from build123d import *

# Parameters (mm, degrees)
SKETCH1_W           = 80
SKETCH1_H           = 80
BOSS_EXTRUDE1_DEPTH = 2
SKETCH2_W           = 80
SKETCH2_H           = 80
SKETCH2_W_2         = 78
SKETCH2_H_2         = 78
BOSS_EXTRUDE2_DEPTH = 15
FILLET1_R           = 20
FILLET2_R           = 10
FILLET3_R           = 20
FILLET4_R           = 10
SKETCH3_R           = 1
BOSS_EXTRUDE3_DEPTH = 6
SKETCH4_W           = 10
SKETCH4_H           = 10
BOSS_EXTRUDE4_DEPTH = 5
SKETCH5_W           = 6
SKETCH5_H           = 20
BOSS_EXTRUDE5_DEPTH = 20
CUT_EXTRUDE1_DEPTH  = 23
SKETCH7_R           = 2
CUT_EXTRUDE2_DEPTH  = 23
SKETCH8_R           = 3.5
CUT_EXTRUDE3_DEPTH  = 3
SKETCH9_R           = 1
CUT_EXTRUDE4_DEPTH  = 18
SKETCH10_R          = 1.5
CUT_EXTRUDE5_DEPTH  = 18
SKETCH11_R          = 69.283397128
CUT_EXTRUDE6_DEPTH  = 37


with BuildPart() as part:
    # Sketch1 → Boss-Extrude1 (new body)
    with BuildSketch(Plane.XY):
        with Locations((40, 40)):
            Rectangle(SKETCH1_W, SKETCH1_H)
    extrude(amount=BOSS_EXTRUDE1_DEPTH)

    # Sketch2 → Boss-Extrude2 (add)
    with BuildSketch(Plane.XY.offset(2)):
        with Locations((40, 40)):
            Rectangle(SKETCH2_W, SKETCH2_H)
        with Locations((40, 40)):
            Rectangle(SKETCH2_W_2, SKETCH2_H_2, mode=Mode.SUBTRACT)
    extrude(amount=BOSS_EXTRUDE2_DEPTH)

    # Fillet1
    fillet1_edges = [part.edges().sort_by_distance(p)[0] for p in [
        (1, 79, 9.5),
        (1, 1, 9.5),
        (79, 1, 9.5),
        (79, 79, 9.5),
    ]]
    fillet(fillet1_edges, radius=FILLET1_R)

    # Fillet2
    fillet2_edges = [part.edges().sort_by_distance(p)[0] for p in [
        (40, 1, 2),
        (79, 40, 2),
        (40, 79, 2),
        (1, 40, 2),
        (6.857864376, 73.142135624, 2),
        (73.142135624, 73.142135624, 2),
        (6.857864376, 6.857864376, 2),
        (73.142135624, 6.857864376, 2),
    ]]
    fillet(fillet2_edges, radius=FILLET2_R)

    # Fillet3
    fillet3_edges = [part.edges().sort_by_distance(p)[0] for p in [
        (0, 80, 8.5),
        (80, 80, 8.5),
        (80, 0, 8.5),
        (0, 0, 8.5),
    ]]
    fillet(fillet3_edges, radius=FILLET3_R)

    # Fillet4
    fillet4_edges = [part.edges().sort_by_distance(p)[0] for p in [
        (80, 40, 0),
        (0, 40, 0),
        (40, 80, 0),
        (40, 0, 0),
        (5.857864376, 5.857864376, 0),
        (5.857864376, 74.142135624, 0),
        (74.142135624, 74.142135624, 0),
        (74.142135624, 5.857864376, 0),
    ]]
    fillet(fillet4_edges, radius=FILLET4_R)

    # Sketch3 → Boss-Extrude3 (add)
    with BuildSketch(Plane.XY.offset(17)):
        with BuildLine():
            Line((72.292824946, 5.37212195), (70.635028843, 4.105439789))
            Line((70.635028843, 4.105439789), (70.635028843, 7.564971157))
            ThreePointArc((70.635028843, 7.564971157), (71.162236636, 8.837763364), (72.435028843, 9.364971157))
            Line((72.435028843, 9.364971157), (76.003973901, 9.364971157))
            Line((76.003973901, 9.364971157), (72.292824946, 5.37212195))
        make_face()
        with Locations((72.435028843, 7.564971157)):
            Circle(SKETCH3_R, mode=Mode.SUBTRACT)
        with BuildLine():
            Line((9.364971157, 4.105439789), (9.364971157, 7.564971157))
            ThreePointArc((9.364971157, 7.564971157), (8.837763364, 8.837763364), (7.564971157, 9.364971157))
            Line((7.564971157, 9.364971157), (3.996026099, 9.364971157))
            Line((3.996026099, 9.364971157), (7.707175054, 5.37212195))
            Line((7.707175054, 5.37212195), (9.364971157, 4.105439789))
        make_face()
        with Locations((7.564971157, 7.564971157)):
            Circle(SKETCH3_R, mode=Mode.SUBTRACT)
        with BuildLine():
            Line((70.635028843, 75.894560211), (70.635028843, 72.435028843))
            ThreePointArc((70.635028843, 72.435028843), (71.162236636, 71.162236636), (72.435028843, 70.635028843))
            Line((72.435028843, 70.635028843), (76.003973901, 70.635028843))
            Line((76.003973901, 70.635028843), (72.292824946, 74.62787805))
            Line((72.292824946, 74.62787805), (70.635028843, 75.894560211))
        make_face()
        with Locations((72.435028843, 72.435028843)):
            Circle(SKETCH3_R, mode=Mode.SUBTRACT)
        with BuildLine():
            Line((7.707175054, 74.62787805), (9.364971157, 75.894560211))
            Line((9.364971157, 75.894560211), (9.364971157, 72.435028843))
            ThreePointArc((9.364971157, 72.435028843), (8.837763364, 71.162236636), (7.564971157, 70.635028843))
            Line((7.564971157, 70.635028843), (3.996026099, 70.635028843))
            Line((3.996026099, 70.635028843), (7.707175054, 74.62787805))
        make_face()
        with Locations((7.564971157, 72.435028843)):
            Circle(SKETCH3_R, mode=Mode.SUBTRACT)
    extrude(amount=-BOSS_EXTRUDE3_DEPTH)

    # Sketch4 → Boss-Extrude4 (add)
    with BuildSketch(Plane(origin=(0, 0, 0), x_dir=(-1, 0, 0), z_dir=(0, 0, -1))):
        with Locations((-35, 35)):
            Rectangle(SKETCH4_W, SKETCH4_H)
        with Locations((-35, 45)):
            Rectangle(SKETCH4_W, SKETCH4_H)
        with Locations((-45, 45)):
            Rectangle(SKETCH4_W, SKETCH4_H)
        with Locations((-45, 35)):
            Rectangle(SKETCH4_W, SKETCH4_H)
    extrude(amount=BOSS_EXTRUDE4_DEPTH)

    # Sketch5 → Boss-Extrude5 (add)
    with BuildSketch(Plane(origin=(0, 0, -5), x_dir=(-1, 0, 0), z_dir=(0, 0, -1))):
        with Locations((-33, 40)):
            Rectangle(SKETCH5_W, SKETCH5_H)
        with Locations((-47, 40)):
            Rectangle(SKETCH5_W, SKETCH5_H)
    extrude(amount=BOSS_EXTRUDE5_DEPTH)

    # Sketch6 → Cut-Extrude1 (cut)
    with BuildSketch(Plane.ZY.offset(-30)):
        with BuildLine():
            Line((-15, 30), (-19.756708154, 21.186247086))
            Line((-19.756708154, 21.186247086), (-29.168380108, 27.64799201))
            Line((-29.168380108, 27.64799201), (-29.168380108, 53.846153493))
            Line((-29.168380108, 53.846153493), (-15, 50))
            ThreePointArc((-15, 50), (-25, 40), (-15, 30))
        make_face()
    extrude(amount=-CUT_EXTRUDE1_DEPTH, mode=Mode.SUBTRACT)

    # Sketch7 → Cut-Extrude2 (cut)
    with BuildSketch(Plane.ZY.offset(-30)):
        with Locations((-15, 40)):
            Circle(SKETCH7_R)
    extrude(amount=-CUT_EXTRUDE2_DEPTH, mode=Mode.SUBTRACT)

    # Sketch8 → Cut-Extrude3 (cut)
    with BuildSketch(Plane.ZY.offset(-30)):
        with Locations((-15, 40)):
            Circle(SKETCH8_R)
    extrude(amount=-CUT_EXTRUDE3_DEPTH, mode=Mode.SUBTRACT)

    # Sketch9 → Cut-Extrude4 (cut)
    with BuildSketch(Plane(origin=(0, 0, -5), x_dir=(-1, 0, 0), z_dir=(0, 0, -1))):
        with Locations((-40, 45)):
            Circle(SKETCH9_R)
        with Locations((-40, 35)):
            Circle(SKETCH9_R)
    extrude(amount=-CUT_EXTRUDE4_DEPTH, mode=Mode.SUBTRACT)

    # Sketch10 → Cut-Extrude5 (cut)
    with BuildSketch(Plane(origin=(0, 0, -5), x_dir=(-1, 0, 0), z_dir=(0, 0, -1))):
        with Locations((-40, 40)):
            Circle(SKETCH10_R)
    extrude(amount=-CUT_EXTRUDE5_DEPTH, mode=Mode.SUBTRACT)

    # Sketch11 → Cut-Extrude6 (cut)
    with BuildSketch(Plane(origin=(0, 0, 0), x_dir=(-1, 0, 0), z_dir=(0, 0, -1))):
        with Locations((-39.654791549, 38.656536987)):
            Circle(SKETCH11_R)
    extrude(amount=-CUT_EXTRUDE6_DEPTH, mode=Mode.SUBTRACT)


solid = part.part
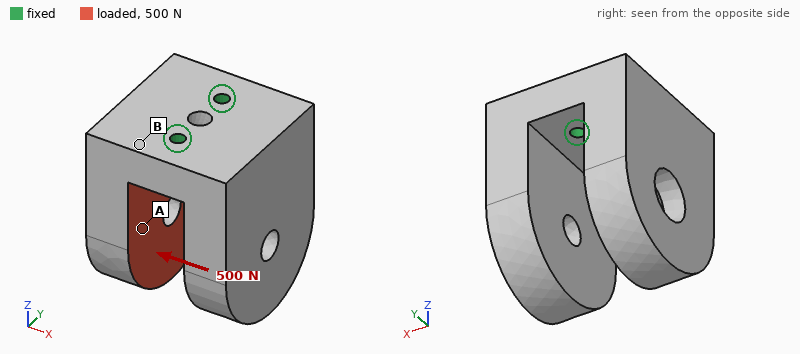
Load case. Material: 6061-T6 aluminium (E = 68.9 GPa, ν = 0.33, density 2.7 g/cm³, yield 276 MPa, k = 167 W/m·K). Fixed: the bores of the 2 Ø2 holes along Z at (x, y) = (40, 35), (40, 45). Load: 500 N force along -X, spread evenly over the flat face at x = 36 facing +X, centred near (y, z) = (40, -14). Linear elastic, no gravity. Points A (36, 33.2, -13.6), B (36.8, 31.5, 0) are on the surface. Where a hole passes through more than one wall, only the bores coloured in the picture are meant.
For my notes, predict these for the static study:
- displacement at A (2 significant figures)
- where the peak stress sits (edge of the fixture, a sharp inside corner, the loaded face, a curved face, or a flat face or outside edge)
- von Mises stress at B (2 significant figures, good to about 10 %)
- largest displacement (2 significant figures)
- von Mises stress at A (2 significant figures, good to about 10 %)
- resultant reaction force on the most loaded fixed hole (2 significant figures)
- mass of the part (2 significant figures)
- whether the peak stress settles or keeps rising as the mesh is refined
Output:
39 µm
edge of the fixture
54 MPa
91 µm
14 MPa
260 N
16 g
keeps rising
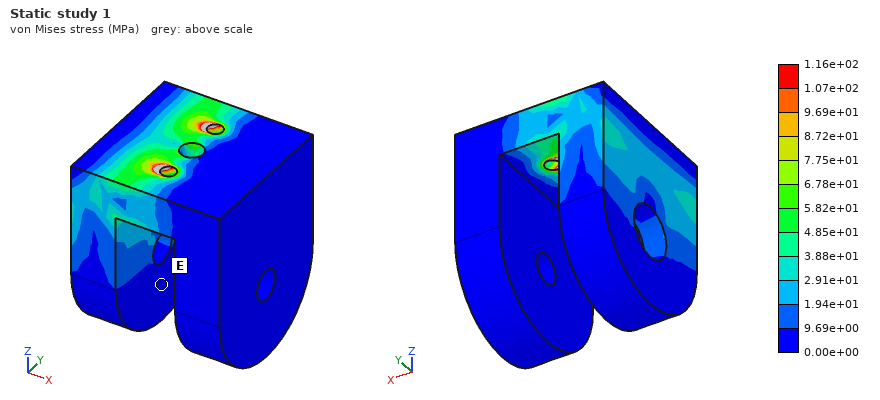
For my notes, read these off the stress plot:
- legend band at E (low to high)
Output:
0.00e+00 to 9.69e+00 MPa
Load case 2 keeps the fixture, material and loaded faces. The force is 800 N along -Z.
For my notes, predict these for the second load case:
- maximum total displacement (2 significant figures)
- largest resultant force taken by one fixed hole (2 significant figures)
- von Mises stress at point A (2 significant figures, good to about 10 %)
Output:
8.6 µm
400 N
16 MPa
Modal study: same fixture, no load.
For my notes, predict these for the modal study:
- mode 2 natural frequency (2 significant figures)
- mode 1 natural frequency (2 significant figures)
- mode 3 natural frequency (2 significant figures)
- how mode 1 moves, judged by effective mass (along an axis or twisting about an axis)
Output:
6700 Hz
5800 Hz
11 kHz
along X
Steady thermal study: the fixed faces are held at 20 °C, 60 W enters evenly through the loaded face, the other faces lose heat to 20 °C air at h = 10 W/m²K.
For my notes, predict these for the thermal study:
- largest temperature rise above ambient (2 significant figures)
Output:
60 K
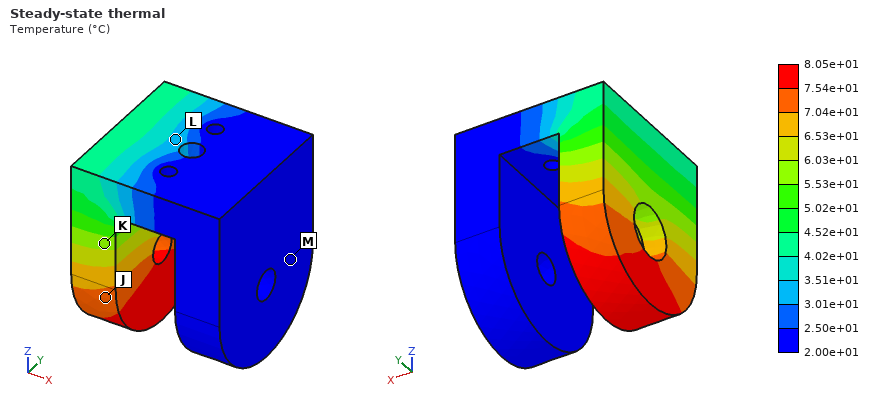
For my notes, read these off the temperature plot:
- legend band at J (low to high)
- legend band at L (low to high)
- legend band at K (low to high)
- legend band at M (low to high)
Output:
7.04e+01 to 7.54e+01 °C
3.01e+01 to 3.51e+01 °C
5.53e+01 to 6.03e+01 °C
2.00e+01 to 2.50e+01 °C
